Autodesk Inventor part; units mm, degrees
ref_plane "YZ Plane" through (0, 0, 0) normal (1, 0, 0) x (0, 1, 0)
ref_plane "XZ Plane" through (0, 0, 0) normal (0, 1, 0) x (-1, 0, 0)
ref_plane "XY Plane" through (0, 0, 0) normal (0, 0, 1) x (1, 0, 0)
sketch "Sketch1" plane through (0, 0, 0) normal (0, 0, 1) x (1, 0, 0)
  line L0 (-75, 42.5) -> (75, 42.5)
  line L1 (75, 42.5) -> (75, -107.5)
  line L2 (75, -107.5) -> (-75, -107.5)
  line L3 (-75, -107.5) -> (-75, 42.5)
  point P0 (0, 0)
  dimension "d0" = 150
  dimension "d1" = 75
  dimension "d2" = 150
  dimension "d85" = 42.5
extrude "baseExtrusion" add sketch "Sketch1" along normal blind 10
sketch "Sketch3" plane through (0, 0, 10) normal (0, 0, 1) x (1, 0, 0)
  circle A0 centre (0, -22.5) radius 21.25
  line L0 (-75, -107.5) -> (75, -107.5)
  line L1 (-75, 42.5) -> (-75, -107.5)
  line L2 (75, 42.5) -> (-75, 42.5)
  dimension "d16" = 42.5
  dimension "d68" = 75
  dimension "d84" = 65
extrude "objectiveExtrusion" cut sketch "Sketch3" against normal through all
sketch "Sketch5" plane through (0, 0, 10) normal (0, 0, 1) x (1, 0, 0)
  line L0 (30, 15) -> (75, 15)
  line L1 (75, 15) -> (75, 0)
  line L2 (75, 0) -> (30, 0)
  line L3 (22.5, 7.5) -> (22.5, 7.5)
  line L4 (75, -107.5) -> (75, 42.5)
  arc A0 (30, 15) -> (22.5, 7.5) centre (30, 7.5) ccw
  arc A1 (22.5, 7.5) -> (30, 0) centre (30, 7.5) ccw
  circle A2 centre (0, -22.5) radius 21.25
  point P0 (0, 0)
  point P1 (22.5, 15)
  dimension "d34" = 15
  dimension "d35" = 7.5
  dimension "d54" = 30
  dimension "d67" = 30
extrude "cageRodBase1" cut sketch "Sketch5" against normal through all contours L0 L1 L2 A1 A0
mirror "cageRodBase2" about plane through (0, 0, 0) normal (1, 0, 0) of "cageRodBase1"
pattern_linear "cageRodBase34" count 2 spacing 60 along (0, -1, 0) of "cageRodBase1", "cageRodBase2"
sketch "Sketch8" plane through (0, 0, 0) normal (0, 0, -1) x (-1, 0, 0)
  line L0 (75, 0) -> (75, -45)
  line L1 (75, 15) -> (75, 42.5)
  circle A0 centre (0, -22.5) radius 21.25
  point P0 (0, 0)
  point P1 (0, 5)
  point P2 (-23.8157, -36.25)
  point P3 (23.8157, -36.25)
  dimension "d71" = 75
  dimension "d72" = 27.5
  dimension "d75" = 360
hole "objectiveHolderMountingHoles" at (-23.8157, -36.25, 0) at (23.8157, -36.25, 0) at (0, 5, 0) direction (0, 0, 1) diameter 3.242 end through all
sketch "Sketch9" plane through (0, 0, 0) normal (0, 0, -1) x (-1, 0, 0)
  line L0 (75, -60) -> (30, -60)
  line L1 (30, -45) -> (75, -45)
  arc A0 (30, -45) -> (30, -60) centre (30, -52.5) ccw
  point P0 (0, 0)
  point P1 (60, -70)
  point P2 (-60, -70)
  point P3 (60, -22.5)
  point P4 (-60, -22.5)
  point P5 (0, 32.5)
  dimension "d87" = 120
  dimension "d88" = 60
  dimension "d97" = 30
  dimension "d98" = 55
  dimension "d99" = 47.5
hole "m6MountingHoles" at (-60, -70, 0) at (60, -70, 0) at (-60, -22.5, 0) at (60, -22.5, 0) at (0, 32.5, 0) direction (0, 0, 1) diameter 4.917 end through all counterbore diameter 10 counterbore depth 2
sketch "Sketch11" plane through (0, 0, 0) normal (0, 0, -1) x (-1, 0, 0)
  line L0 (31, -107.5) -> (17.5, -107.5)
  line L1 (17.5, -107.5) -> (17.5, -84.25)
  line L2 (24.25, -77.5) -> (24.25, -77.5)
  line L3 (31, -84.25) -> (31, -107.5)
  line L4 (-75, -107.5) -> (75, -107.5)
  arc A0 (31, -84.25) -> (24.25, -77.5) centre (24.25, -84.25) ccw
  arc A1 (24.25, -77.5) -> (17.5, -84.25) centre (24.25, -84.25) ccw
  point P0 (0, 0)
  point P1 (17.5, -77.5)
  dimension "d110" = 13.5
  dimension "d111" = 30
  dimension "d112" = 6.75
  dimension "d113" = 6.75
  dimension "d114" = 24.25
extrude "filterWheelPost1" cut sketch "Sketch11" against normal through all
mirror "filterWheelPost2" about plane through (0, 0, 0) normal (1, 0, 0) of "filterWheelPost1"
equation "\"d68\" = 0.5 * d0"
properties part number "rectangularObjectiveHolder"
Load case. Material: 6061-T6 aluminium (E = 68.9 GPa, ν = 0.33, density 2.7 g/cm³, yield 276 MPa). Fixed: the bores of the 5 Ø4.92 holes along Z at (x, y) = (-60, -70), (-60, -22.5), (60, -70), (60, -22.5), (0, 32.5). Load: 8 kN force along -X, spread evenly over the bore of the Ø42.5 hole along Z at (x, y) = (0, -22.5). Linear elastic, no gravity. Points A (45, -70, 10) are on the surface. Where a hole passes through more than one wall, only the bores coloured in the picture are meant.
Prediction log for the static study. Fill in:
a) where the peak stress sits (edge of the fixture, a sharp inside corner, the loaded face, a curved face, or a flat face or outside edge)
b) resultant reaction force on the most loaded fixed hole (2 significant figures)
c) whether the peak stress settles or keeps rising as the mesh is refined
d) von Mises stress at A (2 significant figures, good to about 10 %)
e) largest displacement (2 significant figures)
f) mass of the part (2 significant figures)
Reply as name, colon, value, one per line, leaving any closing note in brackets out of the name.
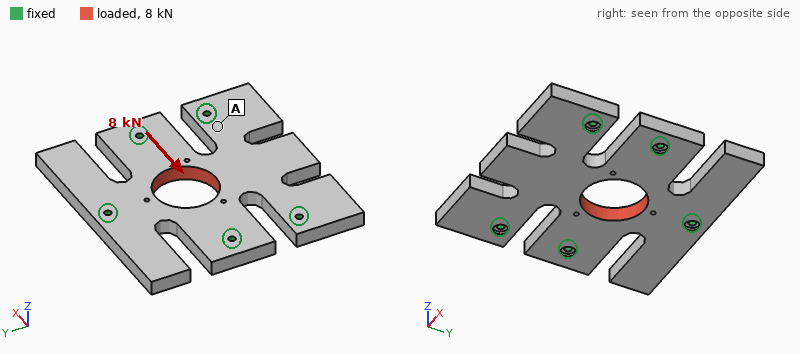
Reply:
where the peak stress sits: edge of the fixture
resultant reaction force on the most loaded fixed hole: 3.0 kN
whether the peak stress settles or keeps rising as the mesh is refined: keeps rising
von Mises stress at A: 4.4 MPa
largest displacement: 20 µm
mass of the part: 460 g
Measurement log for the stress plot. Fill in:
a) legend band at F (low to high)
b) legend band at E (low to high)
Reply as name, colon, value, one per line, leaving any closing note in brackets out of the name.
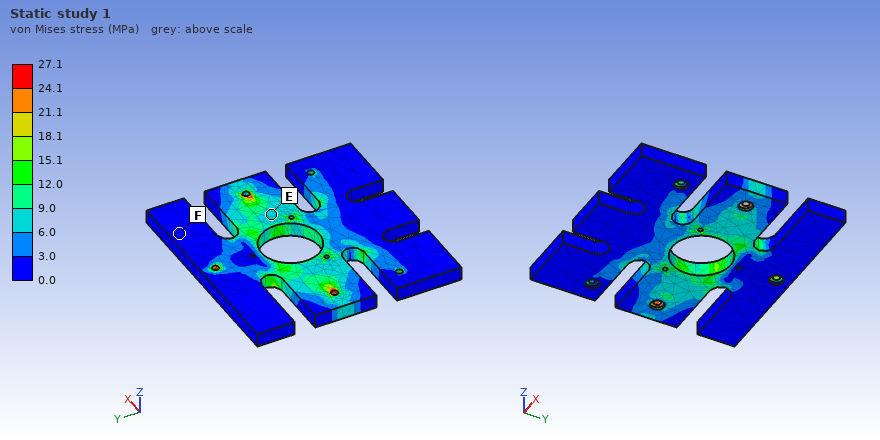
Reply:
legend band at F: 0.0 to 3.0 MPa
legend band at E: 6.0 to 9.0 MPa
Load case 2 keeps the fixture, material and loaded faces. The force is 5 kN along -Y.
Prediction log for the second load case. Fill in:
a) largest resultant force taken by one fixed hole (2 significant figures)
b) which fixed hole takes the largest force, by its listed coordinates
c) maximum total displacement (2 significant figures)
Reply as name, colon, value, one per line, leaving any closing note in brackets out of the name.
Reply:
largest resultant force taken by one fixed hole: 2.9 kN
which fixed hole takes the largest force, by its listed coordinates: (0, 32.5)
maximum total displacement: 14 µm
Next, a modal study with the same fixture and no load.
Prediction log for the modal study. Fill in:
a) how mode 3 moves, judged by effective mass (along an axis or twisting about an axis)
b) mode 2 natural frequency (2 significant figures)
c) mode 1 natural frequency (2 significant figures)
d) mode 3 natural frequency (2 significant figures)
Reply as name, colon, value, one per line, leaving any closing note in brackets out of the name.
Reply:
how mode 3 moves, judged by effective mass: along Z
mode 2 natural frequency: 1600 Hz
mode 1 natural frequency: 1400 Hz
mode 3 natural frequency: 2100 Hz
